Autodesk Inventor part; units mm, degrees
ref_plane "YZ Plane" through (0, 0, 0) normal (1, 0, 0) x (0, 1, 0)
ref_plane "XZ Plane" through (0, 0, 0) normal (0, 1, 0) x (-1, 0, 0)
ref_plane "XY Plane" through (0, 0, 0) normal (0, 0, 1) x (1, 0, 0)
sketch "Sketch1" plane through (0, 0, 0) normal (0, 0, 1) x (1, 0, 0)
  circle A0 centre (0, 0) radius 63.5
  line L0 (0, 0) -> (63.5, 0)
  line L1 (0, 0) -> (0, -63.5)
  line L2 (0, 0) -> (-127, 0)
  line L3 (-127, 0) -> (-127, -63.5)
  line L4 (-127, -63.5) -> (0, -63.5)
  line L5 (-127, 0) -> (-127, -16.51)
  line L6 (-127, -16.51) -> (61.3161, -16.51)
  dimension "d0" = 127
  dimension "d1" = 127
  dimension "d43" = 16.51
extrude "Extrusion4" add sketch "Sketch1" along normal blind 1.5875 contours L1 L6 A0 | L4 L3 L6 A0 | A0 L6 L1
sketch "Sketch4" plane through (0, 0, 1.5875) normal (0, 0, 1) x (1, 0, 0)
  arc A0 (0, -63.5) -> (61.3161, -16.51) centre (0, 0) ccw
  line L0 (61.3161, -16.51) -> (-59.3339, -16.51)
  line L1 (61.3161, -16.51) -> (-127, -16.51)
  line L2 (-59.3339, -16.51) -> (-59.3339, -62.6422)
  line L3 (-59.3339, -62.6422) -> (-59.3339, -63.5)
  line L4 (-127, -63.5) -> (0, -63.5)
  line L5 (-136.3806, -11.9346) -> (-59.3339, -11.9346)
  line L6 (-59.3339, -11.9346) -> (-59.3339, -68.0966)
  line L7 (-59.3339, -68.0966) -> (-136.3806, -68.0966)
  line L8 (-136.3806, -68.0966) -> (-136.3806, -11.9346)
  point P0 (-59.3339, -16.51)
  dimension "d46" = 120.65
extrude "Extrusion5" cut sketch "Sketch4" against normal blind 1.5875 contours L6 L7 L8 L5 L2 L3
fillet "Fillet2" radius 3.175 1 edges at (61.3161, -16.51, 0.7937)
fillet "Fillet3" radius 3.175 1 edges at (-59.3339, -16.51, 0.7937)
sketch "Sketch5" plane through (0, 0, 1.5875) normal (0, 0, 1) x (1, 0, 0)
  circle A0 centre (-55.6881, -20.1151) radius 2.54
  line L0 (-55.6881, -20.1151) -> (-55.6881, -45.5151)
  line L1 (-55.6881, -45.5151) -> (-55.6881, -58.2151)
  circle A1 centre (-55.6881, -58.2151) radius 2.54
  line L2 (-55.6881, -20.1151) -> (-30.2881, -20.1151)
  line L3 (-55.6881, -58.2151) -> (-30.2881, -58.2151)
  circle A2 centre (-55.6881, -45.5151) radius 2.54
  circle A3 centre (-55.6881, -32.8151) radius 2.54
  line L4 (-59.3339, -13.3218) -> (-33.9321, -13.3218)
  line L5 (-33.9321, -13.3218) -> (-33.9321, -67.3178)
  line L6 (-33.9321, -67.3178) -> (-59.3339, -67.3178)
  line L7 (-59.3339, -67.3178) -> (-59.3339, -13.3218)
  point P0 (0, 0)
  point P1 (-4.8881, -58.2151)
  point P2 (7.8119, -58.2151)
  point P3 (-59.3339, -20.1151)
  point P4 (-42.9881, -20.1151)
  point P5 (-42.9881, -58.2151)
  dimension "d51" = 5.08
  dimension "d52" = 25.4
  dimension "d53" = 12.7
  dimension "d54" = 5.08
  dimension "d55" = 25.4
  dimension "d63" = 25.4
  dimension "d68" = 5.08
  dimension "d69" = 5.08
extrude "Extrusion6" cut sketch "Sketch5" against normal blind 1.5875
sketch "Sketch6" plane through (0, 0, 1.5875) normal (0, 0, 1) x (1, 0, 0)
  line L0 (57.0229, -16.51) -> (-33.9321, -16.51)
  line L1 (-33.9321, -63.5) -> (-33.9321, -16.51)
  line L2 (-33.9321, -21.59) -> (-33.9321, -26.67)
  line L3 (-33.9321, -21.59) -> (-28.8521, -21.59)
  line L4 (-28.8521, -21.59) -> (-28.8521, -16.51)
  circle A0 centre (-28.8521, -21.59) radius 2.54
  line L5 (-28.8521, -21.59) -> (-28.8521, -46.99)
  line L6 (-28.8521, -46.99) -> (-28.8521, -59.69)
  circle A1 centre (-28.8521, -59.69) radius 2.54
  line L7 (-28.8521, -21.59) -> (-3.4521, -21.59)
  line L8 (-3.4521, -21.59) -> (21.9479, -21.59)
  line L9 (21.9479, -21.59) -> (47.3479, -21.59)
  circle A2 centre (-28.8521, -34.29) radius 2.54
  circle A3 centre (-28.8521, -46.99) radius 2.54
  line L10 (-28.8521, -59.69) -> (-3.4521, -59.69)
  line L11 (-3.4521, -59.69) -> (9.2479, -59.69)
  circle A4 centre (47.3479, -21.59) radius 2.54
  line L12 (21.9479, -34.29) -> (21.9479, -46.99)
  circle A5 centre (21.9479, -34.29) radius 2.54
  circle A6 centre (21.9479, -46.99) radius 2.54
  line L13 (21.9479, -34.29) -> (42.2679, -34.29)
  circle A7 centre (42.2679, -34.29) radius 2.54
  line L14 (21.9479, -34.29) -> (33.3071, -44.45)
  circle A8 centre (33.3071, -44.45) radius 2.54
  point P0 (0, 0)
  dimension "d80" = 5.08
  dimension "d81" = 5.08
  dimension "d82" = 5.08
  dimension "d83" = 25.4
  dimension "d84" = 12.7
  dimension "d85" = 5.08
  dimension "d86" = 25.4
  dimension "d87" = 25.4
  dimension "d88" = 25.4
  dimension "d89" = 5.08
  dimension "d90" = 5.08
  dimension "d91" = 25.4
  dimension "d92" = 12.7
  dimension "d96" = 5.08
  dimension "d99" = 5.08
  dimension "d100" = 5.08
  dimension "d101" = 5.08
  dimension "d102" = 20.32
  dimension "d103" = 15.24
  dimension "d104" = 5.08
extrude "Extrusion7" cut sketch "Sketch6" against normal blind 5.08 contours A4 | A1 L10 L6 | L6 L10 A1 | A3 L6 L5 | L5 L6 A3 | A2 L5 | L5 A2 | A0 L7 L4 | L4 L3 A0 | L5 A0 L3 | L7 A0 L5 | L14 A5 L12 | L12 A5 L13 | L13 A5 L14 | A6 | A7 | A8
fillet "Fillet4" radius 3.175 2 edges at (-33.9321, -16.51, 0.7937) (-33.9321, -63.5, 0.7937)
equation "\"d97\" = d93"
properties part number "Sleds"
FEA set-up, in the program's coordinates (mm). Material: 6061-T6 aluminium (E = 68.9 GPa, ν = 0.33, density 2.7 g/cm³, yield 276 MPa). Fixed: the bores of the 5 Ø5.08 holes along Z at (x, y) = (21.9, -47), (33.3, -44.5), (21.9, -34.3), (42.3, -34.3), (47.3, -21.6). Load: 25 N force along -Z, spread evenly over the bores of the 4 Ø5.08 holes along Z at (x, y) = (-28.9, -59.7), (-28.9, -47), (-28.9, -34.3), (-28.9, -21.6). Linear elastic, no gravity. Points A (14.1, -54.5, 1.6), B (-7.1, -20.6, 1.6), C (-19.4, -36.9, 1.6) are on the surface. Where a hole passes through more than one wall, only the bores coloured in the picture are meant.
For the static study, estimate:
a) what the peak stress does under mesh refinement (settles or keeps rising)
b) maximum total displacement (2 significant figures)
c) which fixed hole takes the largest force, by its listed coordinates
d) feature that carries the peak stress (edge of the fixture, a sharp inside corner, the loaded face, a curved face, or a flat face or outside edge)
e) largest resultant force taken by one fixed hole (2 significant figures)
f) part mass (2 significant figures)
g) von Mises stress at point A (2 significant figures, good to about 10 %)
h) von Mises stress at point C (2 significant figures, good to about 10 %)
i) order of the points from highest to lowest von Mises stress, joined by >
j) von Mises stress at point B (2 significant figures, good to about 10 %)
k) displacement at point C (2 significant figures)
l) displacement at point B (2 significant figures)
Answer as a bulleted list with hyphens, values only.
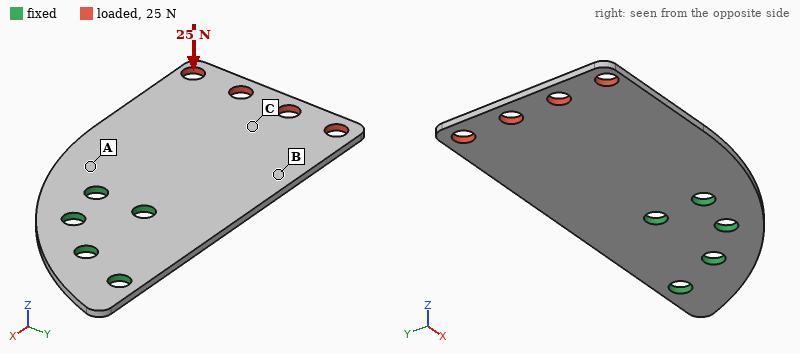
- keeps rising
- 1.1 mm
- (21.9, -34.3)
- edge of the fixture
- 20 N
- 15 g
- 51 MPa
- 11 MPa
- A > B > C
- 28 MPa
- 0.68 mm
- 0.35 mm
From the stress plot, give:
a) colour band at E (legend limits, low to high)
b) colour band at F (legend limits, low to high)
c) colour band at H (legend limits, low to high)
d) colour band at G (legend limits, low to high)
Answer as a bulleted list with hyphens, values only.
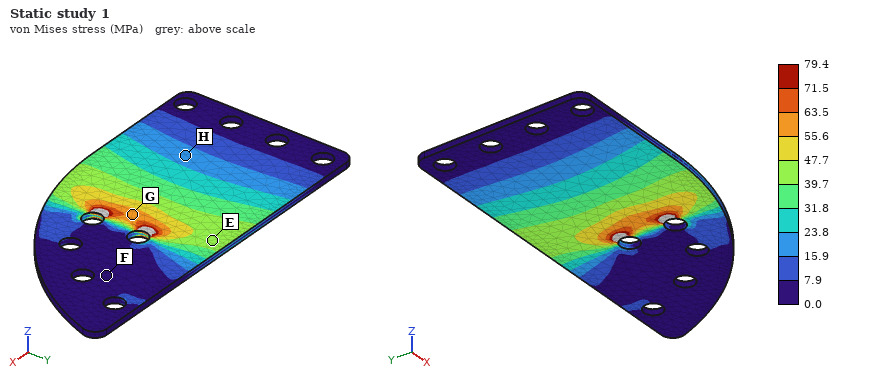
- 39.7 to 47.7 MPa
- 0.0 to 7.9 MPa
- 15.9 to 23.8 MPa
- 55.6 to 63.5 MPa
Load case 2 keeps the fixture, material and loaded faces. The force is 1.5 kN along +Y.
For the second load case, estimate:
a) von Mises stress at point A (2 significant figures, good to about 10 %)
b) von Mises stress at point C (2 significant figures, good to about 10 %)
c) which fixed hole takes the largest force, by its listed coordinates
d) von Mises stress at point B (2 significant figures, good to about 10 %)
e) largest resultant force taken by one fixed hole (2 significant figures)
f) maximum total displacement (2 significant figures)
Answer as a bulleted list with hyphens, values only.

- 82 MPa
- 53 MPa
- (21.9, -47)
- 51 MPa
- 2.7 kN
- 0.23 mm
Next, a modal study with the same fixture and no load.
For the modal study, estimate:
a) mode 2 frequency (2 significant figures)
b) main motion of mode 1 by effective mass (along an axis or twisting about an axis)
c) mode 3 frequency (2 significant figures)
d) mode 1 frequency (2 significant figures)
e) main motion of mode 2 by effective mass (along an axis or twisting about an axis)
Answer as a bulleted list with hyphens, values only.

- 1100 Hz
- along Z
- 2600 Hz
- 460 Hz
- twisting about X
